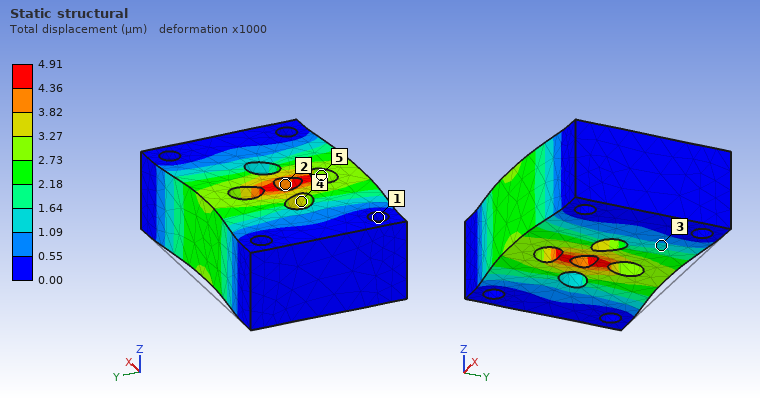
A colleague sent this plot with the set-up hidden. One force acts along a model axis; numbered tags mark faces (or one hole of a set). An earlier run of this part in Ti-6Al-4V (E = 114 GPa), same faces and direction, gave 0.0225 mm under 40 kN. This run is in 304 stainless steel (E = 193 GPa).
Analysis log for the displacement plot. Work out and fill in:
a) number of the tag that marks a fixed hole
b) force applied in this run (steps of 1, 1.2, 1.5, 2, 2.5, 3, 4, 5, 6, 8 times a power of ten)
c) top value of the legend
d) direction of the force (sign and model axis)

1
15 kN
4.91 µm
-Y
